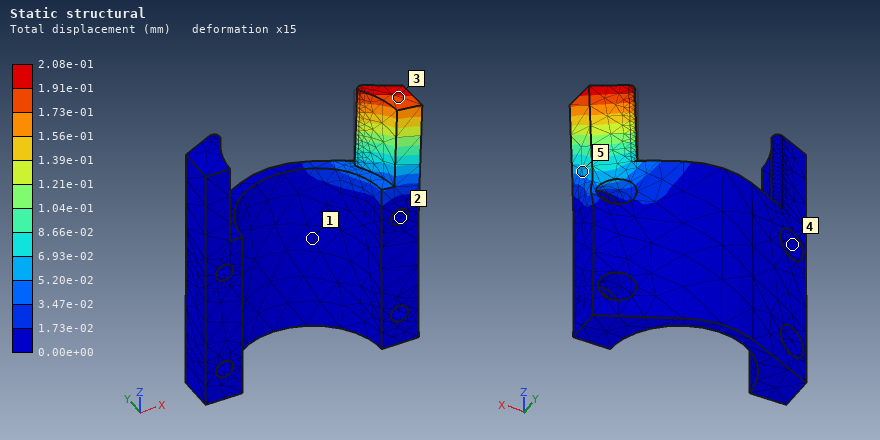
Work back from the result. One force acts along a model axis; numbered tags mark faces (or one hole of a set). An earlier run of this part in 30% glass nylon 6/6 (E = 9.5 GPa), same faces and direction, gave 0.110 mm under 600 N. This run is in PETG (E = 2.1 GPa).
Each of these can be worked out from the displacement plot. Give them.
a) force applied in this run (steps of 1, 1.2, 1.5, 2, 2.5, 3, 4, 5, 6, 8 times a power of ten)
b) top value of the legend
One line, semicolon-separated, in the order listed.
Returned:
250 N; 2.08e-01 mm
